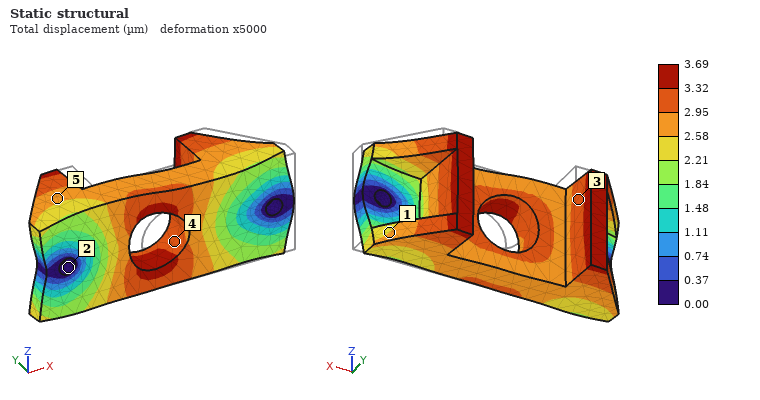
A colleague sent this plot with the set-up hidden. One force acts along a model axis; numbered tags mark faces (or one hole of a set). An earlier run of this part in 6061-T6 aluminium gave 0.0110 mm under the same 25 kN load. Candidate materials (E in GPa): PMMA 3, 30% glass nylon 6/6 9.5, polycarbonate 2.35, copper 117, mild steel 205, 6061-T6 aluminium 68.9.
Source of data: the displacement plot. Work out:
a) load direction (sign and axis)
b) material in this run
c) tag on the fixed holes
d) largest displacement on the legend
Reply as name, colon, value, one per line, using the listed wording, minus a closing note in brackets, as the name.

load direction: -X
material in this run: mild steel
tag on the fixed holes: 2
largest displacement on the legend: 3.69 µm
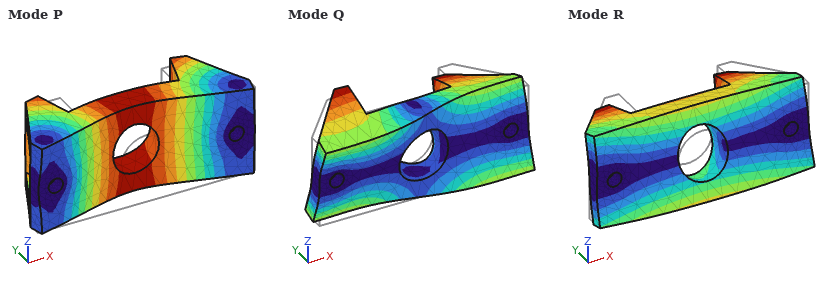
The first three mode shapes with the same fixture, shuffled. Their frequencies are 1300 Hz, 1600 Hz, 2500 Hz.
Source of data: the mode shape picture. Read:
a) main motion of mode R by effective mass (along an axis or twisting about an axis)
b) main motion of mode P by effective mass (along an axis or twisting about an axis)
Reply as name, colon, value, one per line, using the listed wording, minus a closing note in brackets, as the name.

main motion of mode R by effective mass: along Z
main motion of mode P by effective mass: along Y
